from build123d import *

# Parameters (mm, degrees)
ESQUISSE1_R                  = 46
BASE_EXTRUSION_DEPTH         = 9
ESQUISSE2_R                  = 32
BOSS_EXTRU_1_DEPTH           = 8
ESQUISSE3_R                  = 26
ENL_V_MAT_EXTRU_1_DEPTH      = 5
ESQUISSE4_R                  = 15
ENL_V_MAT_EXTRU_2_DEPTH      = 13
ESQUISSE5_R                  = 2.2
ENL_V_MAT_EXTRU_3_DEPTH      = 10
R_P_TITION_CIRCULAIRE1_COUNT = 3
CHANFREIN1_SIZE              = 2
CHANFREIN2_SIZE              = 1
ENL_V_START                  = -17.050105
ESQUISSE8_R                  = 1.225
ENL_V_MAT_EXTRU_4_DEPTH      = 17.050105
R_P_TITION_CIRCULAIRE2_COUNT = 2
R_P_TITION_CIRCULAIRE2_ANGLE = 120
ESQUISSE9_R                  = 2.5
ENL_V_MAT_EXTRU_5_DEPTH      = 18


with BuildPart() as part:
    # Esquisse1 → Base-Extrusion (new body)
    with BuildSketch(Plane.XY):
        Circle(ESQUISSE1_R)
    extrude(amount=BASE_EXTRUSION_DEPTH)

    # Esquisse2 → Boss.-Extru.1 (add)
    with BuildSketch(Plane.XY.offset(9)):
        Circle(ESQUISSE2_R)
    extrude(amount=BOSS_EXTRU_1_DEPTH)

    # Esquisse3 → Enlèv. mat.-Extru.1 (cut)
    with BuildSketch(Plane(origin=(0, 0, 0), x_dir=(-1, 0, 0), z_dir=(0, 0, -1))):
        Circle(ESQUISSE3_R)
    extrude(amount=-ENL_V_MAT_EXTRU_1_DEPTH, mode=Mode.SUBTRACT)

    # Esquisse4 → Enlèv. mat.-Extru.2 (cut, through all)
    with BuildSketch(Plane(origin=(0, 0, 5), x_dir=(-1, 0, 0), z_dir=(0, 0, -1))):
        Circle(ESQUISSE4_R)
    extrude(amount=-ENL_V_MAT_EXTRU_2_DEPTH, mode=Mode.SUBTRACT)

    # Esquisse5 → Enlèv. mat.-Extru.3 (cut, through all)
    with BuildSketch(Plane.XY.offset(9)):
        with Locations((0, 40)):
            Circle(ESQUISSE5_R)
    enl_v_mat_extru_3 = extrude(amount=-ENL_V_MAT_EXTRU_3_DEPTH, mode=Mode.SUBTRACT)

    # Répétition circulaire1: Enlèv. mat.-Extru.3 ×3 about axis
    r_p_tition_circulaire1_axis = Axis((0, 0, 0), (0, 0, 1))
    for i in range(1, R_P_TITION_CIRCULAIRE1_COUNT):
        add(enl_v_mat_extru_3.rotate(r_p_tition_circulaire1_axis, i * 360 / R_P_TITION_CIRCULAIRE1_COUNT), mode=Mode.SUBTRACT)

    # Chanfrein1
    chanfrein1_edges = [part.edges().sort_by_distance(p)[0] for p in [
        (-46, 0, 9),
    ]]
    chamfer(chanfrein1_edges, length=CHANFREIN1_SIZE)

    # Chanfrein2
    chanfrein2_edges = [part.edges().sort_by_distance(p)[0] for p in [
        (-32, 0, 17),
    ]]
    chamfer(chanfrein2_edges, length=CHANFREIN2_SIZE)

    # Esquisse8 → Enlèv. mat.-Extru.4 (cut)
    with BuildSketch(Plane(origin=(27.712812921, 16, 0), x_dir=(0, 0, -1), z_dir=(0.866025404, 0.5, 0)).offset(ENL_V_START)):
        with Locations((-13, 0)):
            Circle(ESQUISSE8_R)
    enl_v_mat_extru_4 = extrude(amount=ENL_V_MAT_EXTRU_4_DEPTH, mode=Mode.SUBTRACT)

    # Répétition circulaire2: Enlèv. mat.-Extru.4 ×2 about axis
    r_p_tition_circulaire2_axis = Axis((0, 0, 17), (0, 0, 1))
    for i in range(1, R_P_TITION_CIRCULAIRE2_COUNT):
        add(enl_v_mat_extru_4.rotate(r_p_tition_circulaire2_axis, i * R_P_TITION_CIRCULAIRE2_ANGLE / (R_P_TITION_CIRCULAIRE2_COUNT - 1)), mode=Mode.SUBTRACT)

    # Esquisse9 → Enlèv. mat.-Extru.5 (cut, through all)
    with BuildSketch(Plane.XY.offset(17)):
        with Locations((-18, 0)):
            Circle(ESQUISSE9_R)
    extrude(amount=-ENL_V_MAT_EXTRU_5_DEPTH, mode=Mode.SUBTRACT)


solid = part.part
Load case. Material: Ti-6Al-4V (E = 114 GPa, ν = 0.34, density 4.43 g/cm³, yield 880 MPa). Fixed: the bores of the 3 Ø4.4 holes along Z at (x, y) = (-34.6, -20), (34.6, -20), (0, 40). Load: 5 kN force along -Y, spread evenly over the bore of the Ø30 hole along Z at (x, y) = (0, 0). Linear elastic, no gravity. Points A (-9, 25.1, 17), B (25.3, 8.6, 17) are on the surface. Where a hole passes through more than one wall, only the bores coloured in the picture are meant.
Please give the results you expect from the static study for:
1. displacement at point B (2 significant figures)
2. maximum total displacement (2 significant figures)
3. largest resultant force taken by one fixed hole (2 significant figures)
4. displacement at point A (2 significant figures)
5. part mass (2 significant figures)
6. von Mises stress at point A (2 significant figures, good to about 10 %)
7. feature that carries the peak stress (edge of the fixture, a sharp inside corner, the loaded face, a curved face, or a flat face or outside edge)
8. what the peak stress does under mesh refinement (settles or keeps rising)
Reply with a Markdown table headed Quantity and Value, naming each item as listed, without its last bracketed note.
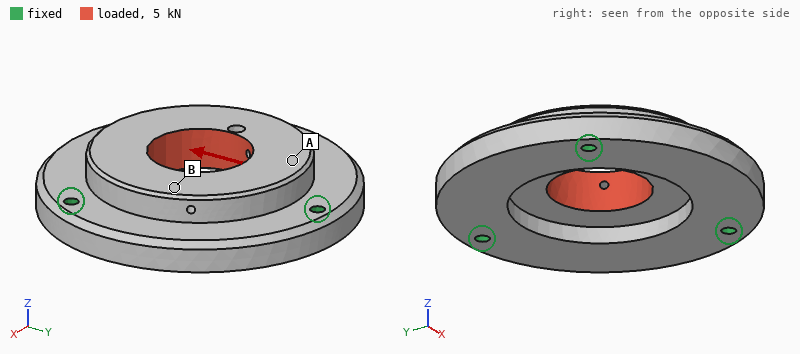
| Quantity | Value |
|---|---|
| displacement at point B | 3.1 µm |
| maximum total displacement | 5.7 µm |
| largest resultant force taken by one fixed hole | 1.7 kN |
| displacement at point A | 2.6 µm |
| part mass | 290 g |
| von Mises stress at point A | 6.3 MPa |
| feature that carries the peak stress | edge of the fixture |
| what the peak stress does under mesh refinement | keeps rising |
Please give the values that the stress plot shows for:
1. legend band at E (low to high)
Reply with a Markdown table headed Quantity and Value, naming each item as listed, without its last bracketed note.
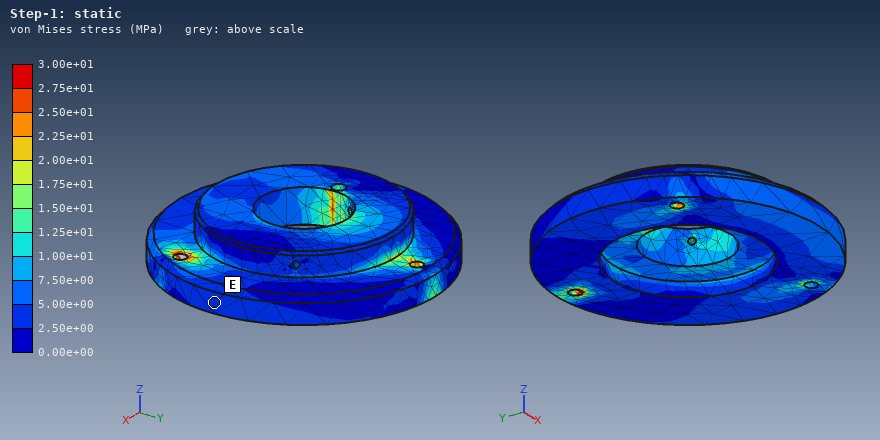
| Quantity | Value |
|---|---|
| legend band at E | 2.50e+00 to 5.00e+00 MPa |
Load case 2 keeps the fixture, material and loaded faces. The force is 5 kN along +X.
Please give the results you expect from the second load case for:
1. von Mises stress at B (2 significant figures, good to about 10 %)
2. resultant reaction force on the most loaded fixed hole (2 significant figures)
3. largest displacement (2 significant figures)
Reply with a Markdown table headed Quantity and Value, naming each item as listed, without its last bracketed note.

| Quantity | Value |
|---|---|
| von Mises stress at B | 4.5 MPa |
| resultant reaction force on the most loaded fixed hole | 1.7 kN |
| largest displacement | 5.5 µm |
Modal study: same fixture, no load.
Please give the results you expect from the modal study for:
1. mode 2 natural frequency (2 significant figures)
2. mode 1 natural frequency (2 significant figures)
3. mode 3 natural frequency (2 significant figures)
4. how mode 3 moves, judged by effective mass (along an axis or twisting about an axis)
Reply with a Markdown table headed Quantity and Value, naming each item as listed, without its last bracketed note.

| Quantity | Value |
|---|---|
| mode 2 natural frequency | 6800 Hz |
| mode 1 natural frequency | 6800 Hz |
| mode 3 natural frequency | 7900 Hz |
| how mode 3 moves, judged by effective mass | along Z |
